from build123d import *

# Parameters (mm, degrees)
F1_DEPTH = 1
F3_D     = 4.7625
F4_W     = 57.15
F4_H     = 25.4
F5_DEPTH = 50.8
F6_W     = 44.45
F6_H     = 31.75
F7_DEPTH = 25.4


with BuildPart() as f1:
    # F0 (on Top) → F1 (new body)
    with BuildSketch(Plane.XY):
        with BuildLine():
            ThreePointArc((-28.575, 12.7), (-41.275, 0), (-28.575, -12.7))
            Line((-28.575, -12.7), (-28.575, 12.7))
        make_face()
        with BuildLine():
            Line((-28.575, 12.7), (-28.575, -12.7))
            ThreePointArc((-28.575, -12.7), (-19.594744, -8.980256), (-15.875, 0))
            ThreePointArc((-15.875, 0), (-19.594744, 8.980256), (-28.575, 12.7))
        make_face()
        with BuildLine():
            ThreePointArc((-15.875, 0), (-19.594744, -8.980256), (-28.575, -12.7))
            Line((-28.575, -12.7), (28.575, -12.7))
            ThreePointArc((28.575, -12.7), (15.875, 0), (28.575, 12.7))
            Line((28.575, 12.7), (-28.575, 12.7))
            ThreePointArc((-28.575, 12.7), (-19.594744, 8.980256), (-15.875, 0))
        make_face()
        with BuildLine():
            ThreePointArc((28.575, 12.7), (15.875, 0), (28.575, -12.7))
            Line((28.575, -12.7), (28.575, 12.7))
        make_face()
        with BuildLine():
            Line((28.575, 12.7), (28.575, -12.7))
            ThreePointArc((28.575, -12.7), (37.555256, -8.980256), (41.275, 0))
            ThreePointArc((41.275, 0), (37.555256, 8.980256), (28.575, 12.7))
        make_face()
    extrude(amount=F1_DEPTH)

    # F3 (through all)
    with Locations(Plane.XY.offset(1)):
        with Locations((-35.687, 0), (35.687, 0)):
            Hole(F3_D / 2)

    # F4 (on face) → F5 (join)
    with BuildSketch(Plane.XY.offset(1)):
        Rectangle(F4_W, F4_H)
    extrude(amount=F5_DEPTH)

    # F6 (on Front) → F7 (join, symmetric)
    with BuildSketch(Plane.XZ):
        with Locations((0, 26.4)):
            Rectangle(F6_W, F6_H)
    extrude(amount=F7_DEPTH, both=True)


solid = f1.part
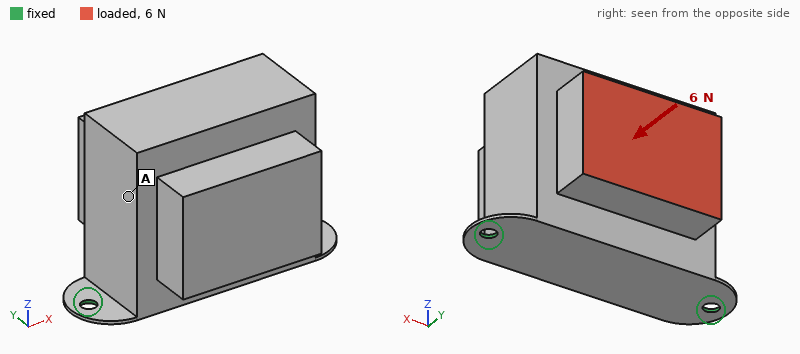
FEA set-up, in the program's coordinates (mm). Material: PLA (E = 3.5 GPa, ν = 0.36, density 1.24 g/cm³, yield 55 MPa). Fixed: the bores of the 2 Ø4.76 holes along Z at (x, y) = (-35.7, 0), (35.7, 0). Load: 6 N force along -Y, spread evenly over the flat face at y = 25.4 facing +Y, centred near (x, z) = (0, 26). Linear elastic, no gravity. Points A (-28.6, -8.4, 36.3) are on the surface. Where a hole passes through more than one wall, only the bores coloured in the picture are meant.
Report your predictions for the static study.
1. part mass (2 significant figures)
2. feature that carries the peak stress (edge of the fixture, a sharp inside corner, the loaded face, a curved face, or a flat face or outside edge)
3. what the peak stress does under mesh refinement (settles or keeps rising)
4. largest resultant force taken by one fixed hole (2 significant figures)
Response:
140 g
edge of the fixture
keeps rising
3.0 N
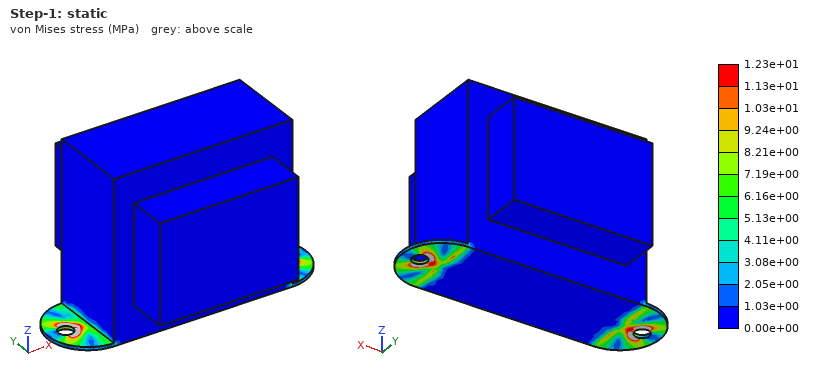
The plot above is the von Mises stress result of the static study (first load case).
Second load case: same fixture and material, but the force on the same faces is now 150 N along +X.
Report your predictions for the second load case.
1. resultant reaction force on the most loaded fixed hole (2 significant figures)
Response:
110 N
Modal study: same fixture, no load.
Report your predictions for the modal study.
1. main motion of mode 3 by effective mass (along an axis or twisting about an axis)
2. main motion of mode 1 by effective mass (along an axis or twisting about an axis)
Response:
along Z
along Y
